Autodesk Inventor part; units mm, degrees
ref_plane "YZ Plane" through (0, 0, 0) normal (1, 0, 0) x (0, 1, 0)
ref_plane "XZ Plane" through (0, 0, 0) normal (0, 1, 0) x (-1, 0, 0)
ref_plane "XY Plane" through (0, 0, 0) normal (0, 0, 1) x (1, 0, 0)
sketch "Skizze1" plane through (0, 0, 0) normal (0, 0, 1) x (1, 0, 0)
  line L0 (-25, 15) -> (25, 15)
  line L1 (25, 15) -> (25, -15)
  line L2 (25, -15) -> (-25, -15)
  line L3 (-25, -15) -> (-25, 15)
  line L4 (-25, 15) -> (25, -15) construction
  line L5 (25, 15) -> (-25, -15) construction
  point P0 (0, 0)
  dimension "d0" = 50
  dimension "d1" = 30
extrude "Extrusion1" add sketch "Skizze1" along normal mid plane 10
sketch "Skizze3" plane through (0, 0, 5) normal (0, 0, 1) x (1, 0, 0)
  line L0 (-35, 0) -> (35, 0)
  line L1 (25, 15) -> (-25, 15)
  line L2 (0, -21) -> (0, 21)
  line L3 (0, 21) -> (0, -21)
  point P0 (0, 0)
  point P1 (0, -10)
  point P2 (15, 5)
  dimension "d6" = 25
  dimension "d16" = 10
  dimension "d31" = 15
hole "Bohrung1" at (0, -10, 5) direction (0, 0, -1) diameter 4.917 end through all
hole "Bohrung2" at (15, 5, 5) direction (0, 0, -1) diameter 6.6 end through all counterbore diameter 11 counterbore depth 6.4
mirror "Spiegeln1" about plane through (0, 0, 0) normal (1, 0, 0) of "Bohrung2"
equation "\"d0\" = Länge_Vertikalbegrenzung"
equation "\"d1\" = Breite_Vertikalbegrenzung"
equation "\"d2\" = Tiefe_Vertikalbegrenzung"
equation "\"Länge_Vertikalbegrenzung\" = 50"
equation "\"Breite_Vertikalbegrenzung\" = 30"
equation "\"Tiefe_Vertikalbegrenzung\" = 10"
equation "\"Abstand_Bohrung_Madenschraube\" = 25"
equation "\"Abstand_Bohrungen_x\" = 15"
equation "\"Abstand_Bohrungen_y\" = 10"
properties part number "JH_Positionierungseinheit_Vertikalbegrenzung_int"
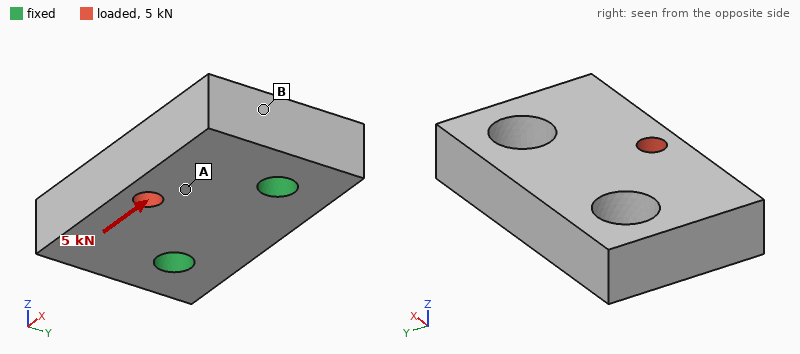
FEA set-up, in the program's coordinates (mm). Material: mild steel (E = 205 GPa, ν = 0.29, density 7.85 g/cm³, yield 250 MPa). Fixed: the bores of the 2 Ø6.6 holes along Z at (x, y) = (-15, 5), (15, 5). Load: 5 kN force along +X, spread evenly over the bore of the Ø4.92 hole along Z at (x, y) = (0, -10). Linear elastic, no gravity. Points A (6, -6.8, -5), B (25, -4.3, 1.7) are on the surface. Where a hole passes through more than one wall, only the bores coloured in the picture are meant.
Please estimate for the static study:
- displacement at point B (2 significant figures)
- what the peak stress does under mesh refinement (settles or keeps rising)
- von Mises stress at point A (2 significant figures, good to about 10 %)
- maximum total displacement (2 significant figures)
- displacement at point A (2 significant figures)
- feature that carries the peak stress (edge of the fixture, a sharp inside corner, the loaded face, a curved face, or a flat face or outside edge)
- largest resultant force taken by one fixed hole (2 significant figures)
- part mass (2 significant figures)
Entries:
3.9 µm
keeps rising
35 MPa
6.0 µm
3.6 µm
edge of the fixture
3.3 kN
100 g
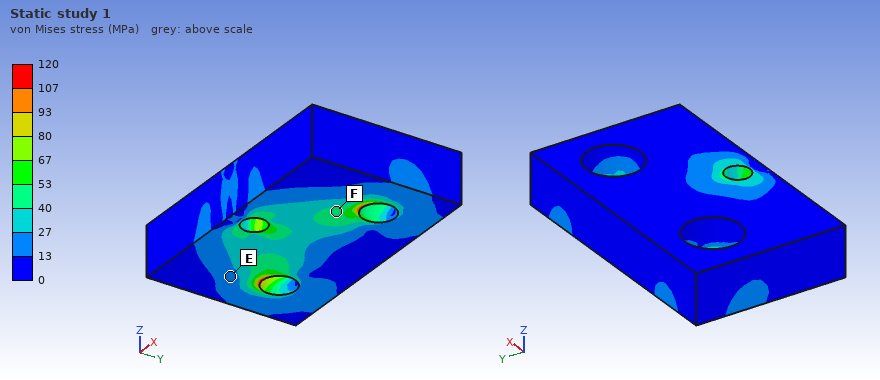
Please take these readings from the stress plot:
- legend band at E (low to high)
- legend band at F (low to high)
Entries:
13 to 27 MPa
40 to 53 MPa
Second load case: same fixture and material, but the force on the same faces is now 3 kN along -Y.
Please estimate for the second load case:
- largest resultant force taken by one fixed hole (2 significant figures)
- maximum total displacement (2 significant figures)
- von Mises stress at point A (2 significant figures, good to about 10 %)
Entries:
1.5 kN
8.7 µm
17 MPa
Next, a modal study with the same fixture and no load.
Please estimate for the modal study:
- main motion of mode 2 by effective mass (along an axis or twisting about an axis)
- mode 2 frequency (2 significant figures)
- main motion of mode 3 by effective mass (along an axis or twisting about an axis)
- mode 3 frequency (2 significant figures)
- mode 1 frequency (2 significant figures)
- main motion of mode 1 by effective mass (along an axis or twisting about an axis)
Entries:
twisting about Y
15 kHz
along X
22 kHz
8100 Hz
along Z
